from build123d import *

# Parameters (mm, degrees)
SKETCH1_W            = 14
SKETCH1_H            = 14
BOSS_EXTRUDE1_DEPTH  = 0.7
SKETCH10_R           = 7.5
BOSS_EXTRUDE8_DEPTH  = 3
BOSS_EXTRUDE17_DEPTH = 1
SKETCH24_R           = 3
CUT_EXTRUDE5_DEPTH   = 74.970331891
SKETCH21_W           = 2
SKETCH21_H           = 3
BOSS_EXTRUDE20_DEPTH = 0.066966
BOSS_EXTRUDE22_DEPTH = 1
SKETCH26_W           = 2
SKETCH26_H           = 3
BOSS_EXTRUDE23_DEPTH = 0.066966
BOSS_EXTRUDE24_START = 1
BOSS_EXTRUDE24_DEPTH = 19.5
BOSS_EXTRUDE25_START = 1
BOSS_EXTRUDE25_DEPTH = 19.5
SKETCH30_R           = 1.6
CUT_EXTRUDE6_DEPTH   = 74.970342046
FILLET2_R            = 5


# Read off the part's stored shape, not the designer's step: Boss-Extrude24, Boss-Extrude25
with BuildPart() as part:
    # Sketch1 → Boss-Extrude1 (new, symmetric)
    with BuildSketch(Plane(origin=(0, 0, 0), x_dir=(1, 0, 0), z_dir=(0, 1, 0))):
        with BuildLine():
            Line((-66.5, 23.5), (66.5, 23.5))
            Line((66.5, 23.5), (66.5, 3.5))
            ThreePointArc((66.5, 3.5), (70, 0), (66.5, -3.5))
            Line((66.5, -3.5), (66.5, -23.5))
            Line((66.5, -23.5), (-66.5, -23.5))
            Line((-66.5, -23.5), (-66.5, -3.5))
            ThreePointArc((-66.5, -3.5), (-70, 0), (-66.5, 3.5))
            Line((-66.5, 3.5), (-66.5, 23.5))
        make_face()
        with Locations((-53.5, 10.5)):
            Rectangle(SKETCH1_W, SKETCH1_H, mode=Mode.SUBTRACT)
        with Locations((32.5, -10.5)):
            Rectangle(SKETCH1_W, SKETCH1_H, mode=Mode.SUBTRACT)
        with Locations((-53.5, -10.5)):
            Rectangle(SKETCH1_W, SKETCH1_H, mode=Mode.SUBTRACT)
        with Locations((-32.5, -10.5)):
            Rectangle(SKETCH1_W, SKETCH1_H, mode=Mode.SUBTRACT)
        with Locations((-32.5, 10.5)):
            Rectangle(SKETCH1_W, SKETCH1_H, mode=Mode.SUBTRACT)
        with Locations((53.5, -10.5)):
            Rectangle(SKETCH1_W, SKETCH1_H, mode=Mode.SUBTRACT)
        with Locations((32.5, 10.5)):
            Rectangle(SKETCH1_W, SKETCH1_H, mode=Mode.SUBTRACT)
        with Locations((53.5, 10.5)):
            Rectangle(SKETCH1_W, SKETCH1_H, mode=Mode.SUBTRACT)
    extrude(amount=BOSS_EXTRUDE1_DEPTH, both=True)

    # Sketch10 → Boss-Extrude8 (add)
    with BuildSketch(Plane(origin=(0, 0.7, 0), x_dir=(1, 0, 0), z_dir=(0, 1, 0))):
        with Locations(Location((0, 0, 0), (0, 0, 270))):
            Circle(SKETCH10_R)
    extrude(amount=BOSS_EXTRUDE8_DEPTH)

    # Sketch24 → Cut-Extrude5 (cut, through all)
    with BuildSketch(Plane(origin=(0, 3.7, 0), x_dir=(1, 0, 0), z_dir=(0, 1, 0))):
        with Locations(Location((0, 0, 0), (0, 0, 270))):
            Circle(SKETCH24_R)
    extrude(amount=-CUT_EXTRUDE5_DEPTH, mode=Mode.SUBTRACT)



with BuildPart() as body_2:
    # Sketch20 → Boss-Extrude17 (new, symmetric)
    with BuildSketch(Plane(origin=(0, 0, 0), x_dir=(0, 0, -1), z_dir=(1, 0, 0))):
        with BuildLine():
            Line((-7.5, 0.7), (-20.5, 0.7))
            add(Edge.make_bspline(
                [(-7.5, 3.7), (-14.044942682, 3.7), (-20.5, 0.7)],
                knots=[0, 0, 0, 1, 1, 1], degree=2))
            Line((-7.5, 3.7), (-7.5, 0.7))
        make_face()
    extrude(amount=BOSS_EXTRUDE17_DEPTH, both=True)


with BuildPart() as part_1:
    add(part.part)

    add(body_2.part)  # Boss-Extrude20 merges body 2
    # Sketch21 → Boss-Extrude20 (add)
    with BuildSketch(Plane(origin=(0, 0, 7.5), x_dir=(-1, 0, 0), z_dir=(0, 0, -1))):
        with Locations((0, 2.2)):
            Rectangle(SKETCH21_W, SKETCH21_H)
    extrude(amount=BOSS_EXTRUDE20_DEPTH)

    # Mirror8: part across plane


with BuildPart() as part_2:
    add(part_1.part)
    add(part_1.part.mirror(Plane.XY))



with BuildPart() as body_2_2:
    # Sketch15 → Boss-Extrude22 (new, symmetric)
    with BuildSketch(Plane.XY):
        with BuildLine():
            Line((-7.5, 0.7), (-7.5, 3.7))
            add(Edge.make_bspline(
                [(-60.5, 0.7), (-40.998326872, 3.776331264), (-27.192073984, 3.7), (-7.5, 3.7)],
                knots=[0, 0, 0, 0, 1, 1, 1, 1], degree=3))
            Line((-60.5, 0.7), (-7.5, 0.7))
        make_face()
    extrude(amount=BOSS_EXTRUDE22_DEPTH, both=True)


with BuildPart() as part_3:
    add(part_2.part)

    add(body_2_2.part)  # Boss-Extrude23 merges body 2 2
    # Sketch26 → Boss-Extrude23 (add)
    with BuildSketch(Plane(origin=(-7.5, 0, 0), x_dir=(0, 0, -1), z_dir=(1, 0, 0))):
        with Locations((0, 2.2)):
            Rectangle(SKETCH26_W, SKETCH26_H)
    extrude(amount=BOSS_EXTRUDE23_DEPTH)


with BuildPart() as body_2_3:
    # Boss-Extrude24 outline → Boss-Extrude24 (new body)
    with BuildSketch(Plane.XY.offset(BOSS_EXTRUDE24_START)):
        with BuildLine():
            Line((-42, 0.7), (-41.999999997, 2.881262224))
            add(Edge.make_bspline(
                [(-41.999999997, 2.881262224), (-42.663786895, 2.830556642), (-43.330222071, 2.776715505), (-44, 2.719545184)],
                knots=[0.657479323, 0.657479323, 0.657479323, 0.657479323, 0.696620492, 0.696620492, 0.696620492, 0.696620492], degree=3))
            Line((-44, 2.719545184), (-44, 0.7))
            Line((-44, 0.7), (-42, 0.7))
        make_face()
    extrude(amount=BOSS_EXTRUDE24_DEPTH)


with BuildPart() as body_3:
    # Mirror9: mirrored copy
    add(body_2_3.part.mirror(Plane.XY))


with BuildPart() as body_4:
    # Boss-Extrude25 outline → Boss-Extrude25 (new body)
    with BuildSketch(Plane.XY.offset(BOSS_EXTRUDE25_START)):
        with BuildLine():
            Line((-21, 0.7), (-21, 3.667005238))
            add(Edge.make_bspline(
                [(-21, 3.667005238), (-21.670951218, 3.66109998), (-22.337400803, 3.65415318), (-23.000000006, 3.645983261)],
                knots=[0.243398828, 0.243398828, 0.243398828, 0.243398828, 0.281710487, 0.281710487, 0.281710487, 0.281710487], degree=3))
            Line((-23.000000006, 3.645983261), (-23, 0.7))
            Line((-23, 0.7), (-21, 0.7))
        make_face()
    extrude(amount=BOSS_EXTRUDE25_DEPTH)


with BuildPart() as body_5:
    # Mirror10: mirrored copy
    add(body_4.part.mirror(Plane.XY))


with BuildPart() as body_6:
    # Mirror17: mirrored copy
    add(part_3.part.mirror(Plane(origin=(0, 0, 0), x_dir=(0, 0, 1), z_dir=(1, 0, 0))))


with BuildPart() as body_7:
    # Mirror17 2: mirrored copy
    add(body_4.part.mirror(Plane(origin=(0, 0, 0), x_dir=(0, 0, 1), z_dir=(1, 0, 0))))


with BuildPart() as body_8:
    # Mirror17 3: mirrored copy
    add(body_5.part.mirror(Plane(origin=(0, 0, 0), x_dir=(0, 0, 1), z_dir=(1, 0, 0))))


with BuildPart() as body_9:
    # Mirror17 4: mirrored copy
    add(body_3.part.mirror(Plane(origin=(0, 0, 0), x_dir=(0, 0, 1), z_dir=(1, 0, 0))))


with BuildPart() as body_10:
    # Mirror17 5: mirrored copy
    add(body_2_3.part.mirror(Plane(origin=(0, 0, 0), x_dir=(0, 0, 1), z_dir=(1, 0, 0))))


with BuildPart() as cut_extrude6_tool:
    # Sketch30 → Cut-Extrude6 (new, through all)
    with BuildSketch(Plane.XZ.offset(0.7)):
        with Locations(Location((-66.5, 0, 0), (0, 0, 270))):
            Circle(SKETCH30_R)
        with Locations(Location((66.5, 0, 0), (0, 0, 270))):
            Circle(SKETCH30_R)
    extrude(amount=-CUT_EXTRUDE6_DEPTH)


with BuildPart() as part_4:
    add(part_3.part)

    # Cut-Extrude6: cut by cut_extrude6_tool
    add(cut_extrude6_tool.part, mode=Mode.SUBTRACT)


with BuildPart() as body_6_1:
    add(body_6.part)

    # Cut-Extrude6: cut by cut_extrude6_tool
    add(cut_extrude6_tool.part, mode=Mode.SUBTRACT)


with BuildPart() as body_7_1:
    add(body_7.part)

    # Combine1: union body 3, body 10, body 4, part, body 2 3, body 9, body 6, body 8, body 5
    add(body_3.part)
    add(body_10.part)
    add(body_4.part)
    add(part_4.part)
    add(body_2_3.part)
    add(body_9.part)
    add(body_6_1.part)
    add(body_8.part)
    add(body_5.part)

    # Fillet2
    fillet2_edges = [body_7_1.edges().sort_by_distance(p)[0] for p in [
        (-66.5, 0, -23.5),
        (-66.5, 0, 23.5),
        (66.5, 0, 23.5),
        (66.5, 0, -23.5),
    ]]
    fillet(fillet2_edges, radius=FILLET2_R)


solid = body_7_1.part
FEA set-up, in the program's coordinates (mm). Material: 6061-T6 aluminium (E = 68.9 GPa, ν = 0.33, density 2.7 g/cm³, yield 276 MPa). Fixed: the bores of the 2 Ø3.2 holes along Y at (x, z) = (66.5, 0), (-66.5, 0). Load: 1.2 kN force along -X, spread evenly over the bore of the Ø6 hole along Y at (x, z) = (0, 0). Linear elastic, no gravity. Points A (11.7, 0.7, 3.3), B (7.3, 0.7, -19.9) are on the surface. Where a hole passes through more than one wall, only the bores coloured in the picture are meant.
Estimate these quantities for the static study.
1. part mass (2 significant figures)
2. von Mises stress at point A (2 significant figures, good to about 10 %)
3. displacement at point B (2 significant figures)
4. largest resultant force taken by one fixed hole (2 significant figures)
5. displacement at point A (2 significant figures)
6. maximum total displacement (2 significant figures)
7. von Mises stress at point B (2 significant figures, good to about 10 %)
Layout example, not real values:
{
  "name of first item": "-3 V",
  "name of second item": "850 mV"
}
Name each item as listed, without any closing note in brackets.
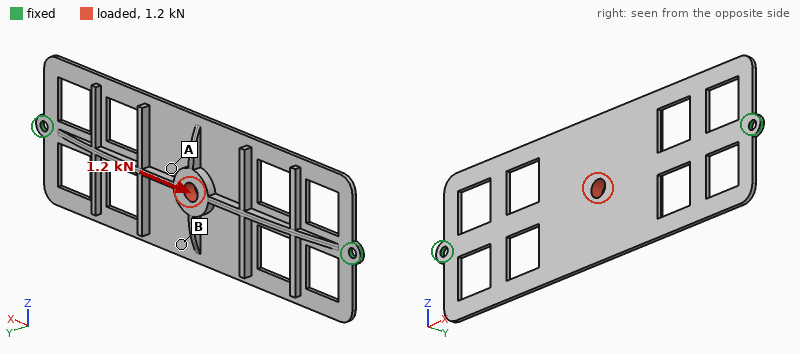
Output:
{
  "part mass": "23 g",
  "von Mises stress at point A": "20 MPa",
  "displacement at point B": "31 µm",
  "largest resultant force taken by one fixed hole": "600 N",
  "displacement at point A": "39 µm",
  "maximum total displacement": "43 µm",
  "von Mises stress at point B": "6.6 MPa"
}
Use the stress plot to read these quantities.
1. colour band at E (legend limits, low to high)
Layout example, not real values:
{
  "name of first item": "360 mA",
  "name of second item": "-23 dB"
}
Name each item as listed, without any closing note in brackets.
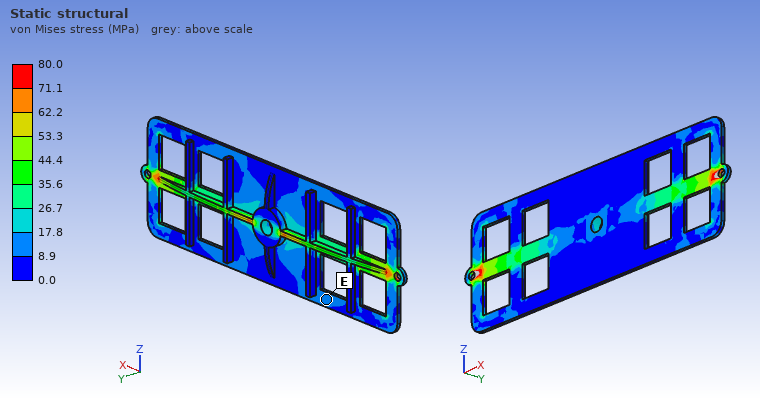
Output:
{
  "colour band at E": "8.9 to 17.8 MPa"
}
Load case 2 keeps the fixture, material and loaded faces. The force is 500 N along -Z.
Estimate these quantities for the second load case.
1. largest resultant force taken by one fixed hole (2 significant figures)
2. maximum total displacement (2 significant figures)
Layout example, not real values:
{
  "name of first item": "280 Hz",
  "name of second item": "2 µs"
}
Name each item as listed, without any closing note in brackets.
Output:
{
  "largest resultant force taken by one fixed hole": "250 N",
  "maximum total displacement": "0.62 mm"
}
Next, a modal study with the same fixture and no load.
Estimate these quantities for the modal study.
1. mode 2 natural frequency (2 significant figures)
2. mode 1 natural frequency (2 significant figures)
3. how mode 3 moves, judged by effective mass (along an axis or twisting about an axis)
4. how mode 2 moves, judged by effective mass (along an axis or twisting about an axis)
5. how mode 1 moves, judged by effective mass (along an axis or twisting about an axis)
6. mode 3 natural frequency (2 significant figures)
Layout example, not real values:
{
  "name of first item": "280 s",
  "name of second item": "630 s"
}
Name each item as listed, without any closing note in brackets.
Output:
{
  "mode 2 natural frequency": "510 Hz",
  "mode 1 natural frequency": "440 Hz",
  "how mode 3 moves, judged by effective mass": "twisting about Z",
  "how mode 2 moves, judged by effective mass": "twisting about X",
  "how mode 1 moves, judged by effective mass": "along Y",
  "mode 3 natural frequency": "1300 Hz"
}
